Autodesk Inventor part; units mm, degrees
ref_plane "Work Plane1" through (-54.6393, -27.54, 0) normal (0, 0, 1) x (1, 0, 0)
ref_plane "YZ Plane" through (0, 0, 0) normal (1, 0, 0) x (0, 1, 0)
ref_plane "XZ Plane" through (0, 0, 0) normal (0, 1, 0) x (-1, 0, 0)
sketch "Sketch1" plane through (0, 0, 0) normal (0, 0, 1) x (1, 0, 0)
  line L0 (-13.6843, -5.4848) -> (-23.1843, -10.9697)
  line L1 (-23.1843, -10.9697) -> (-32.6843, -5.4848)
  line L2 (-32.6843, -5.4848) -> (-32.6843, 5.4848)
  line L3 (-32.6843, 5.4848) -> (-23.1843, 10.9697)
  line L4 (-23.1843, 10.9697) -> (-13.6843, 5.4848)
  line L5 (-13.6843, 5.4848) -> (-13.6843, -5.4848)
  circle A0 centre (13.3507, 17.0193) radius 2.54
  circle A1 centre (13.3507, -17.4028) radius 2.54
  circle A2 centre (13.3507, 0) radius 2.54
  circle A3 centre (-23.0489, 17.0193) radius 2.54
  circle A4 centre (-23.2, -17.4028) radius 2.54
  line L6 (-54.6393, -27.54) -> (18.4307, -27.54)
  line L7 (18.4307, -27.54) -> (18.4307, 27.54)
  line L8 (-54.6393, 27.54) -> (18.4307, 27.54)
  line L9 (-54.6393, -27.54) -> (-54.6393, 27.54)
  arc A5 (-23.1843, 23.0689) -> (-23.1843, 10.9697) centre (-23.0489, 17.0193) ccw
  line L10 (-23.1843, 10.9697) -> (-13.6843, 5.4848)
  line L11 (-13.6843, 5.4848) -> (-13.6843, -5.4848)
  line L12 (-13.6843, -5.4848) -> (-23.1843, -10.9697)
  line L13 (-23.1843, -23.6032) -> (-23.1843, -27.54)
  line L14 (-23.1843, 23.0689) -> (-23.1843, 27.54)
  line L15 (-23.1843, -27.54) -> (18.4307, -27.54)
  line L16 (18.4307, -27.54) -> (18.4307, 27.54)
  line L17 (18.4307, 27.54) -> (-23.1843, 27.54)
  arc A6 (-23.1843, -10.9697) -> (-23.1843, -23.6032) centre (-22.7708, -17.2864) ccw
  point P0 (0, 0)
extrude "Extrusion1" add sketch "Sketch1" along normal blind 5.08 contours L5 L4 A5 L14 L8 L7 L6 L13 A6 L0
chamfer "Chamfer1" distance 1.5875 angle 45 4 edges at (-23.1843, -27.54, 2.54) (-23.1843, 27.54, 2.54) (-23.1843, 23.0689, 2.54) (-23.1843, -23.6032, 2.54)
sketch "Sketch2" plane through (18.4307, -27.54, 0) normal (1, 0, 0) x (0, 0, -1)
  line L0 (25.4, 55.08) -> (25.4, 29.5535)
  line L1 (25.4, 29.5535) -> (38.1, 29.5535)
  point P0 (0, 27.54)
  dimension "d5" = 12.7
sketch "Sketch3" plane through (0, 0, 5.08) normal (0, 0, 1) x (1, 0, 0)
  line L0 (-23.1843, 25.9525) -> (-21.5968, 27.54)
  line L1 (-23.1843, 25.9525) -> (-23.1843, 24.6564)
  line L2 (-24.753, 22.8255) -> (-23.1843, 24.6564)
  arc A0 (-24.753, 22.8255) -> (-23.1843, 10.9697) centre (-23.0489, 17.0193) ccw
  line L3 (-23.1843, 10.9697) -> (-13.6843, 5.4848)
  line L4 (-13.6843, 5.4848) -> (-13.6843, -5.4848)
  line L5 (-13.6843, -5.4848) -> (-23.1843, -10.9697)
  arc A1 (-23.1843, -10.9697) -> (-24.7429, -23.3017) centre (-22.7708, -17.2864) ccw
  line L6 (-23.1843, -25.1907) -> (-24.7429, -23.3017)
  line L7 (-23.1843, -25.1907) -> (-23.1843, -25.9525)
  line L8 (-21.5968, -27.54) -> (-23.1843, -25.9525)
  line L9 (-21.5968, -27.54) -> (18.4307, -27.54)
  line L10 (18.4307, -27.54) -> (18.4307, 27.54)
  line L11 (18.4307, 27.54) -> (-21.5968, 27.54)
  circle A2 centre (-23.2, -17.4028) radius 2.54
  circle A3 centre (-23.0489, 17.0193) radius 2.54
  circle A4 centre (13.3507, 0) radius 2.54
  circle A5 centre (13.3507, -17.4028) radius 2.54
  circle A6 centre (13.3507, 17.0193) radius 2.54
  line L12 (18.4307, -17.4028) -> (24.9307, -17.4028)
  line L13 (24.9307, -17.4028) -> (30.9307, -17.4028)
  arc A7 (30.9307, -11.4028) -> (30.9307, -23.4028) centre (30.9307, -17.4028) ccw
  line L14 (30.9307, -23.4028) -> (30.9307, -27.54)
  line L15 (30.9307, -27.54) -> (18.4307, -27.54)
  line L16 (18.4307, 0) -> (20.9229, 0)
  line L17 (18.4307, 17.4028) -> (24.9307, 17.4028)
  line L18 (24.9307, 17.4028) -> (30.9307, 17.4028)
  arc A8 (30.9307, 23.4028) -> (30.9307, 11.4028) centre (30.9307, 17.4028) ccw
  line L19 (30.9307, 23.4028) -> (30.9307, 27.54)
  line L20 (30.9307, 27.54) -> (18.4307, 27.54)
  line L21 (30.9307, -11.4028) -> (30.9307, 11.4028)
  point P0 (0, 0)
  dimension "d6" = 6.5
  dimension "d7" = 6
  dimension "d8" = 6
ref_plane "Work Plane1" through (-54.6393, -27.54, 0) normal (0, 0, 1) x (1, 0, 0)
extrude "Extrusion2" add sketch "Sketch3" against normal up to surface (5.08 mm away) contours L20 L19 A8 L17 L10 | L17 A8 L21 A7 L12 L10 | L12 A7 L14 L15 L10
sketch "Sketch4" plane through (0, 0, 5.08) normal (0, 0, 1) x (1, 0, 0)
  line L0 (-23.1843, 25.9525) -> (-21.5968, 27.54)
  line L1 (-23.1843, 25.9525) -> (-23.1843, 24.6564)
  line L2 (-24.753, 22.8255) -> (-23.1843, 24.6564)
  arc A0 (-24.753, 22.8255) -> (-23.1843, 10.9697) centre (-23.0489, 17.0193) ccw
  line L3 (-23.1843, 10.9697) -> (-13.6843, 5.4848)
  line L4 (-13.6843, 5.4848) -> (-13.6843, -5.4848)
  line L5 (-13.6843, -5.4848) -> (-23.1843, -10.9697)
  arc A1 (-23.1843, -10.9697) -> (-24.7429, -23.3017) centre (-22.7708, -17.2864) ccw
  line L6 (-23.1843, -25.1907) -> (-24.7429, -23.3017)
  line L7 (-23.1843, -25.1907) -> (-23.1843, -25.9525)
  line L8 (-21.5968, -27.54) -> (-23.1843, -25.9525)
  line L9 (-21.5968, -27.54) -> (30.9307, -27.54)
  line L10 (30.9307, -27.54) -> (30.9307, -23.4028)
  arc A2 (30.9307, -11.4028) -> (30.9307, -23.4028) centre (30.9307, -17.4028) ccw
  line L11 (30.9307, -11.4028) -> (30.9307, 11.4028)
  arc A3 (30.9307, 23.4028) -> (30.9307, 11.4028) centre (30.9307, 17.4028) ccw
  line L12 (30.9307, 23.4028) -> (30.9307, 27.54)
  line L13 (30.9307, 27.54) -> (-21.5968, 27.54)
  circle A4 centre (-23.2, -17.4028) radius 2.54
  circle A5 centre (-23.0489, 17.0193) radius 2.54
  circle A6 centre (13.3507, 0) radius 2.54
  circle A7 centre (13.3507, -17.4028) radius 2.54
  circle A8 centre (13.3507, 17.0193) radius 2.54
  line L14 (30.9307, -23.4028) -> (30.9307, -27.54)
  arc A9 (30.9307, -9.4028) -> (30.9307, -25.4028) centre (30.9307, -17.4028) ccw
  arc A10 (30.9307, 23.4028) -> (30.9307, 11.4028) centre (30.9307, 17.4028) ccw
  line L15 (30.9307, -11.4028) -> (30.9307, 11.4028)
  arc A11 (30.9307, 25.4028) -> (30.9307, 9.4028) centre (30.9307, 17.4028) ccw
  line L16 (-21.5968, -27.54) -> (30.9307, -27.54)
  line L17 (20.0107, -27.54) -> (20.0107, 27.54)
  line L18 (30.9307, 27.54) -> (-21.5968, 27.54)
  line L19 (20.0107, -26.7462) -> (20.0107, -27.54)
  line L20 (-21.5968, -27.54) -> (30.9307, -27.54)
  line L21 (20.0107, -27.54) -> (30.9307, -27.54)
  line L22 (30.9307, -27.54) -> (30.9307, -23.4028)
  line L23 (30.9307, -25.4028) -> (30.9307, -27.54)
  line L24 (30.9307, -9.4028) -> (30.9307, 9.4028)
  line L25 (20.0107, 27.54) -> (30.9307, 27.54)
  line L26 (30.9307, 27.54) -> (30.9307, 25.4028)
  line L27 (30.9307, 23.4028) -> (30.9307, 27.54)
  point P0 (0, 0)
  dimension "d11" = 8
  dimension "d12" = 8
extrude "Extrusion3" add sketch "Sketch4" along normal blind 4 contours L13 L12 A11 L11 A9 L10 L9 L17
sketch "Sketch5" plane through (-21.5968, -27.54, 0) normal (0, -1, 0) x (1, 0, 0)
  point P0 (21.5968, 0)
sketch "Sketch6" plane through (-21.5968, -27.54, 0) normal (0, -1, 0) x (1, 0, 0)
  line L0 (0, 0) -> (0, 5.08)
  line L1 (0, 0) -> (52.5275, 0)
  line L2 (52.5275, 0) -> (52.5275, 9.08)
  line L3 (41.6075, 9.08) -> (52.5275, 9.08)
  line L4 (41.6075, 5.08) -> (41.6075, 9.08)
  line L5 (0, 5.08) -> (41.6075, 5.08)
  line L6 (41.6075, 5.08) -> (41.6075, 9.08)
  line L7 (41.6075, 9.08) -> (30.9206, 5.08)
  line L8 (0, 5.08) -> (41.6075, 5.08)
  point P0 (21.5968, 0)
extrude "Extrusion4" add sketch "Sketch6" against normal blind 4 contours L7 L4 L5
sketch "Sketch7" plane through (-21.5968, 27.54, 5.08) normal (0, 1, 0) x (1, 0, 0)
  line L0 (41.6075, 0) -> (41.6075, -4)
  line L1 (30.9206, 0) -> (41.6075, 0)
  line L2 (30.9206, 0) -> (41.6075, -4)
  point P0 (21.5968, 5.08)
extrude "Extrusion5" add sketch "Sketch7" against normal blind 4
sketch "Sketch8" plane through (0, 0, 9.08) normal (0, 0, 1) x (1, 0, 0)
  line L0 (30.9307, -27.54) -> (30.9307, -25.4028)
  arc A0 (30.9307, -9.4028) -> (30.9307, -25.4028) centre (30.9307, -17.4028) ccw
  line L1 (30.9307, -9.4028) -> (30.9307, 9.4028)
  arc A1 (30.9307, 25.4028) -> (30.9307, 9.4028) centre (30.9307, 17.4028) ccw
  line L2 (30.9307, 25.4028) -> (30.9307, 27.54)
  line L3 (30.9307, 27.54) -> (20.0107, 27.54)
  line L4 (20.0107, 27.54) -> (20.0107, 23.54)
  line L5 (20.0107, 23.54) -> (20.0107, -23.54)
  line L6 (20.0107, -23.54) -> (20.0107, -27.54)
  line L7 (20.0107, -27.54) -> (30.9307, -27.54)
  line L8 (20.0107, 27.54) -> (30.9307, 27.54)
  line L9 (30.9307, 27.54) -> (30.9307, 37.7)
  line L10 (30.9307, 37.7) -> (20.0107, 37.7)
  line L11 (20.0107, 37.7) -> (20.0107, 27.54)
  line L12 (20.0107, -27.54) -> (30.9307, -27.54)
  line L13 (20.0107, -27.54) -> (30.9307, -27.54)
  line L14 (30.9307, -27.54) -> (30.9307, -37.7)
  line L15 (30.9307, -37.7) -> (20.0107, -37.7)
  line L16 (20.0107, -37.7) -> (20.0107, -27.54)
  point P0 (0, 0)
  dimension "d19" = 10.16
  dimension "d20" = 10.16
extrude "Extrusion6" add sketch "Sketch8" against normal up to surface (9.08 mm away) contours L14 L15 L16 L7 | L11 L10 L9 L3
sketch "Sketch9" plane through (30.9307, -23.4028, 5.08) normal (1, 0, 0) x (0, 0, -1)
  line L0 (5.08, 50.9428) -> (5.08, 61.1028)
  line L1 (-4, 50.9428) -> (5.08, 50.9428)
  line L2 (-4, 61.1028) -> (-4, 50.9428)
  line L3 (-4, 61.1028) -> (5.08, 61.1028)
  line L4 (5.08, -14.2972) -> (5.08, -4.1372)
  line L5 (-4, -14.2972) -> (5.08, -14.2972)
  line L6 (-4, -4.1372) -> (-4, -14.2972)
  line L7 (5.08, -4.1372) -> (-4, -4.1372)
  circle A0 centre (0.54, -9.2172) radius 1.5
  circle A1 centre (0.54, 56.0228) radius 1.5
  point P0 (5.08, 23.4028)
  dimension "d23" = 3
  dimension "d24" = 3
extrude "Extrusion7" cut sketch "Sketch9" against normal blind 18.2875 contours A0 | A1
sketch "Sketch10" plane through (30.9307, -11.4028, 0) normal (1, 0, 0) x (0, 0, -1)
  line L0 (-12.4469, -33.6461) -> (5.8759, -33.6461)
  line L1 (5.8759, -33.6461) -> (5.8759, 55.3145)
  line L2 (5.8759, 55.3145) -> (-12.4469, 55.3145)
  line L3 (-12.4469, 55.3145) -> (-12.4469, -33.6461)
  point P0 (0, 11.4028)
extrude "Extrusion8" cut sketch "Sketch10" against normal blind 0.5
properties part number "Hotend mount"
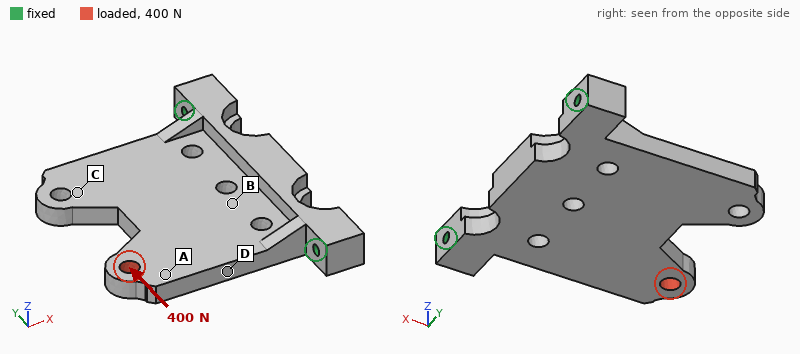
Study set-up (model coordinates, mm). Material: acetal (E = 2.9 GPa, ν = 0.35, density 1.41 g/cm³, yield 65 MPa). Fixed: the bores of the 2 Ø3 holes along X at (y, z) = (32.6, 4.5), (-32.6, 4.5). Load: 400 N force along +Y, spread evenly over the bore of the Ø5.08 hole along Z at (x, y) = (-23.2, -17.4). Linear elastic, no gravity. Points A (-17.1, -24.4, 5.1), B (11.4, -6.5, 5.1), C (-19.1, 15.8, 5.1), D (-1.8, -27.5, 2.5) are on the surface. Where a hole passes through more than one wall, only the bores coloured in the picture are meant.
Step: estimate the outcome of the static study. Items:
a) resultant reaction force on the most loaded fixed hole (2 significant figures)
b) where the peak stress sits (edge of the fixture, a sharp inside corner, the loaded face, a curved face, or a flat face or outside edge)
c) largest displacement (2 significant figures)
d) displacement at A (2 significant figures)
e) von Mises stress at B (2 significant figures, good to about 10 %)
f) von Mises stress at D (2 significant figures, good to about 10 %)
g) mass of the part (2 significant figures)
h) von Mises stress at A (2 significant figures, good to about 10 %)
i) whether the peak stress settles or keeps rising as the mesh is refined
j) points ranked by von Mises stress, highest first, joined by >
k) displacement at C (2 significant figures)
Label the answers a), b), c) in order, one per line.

a) 410 N
b) edge of the fixture
c) 0.43 mm
d) 0.31 mm
e) 3.7 MPa
f) 9.5 MPa
g) 24 g
h) 6.0 MPa
i) keeps rising
j) D > A > B > C
k) 0.18 mm
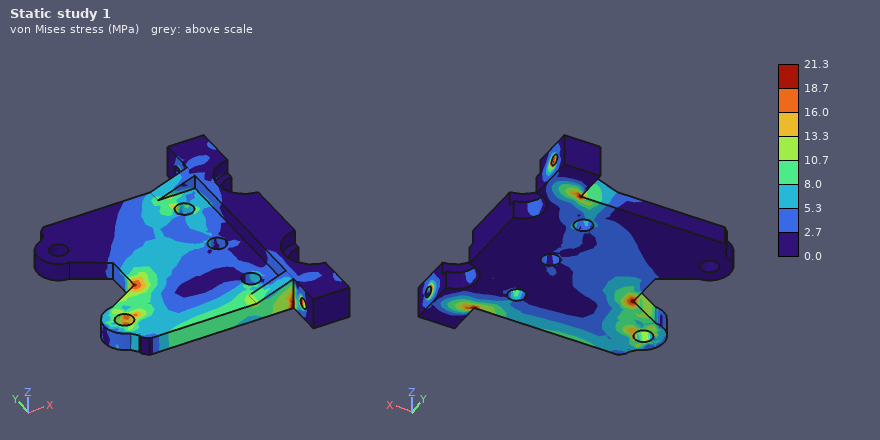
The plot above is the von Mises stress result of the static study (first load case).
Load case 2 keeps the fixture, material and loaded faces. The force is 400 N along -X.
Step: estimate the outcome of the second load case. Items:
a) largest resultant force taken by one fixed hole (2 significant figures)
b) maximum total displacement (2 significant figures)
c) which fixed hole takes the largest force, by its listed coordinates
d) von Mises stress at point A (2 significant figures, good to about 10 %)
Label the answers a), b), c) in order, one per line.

a) 340 N
b) 0.31 mm
c) (-32.6, 4.5)
d) 3.9 MPa
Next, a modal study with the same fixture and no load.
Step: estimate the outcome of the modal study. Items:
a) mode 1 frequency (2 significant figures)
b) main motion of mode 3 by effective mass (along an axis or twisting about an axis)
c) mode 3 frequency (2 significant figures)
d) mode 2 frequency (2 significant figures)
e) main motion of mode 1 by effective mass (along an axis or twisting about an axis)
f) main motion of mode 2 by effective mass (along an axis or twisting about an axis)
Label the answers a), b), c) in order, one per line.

a) 430 Hz
b) along Z
c) 1800 Hz
d) 990 Hz
e) along Z
f) twisting about X
